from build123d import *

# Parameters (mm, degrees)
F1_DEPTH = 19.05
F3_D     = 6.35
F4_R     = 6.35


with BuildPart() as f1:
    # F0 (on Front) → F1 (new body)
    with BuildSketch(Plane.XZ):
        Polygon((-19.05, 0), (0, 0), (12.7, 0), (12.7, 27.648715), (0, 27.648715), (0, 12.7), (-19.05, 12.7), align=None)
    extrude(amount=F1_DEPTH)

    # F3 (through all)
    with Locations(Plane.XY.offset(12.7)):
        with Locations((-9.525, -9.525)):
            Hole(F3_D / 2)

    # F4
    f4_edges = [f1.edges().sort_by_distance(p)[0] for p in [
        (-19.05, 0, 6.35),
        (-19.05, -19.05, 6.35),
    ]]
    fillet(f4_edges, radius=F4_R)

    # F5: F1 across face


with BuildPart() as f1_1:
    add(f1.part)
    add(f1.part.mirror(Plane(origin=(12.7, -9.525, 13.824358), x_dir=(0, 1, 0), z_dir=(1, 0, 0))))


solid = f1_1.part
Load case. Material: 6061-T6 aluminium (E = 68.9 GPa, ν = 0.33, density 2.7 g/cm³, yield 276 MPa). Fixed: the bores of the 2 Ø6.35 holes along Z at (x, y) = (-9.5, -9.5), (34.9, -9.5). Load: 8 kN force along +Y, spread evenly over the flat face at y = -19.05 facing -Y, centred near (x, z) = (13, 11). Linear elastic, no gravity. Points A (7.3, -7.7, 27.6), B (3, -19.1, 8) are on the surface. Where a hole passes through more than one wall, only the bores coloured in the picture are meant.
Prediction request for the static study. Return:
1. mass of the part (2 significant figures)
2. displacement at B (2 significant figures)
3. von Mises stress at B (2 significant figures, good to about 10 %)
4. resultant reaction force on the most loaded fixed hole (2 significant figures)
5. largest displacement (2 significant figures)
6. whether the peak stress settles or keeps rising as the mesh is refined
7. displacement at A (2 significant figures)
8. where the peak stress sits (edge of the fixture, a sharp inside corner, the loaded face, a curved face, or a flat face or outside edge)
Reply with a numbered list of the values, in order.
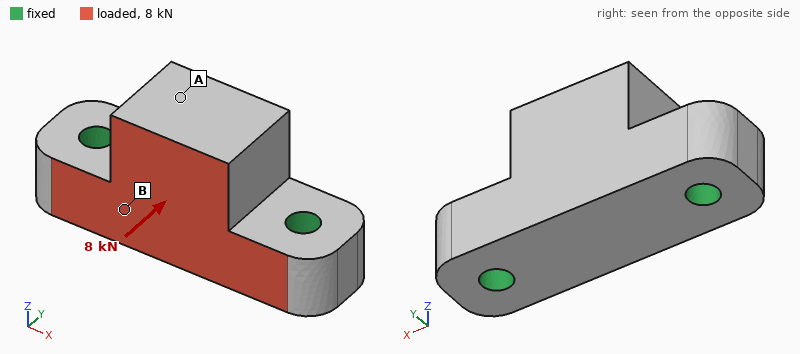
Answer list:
1. 58 g
2. 16 µm
3. 40 MPa
4. 4.0 kN
5. 45 µm
6. keeps rising
7. 42 µm
8. edge of the fixture
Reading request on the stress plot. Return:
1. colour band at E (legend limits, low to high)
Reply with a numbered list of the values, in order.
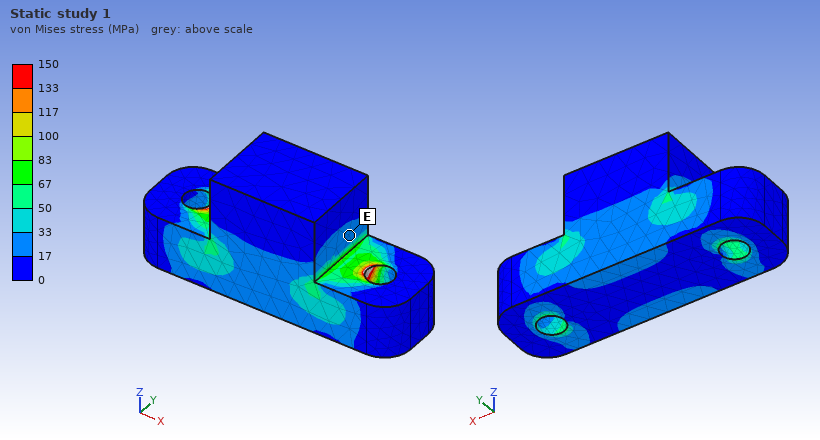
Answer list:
1. 17 to 33 MPa
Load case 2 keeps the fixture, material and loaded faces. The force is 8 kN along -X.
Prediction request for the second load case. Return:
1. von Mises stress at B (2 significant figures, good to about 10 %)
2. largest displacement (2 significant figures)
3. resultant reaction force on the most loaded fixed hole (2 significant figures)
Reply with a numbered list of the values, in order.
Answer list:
1. 21 MPa
2. 18 µm
3. 4.4 kN
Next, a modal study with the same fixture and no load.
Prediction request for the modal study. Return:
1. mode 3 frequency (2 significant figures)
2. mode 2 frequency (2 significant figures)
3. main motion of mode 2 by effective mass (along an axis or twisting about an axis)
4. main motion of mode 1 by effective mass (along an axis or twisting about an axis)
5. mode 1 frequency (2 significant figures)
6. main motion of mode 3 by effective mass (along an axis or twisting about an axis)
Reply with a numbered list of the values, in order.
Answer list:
1. 23 kHz
2. 20 kHz
3. along Z
4. along Y
5. 11 kHz
6. along X
